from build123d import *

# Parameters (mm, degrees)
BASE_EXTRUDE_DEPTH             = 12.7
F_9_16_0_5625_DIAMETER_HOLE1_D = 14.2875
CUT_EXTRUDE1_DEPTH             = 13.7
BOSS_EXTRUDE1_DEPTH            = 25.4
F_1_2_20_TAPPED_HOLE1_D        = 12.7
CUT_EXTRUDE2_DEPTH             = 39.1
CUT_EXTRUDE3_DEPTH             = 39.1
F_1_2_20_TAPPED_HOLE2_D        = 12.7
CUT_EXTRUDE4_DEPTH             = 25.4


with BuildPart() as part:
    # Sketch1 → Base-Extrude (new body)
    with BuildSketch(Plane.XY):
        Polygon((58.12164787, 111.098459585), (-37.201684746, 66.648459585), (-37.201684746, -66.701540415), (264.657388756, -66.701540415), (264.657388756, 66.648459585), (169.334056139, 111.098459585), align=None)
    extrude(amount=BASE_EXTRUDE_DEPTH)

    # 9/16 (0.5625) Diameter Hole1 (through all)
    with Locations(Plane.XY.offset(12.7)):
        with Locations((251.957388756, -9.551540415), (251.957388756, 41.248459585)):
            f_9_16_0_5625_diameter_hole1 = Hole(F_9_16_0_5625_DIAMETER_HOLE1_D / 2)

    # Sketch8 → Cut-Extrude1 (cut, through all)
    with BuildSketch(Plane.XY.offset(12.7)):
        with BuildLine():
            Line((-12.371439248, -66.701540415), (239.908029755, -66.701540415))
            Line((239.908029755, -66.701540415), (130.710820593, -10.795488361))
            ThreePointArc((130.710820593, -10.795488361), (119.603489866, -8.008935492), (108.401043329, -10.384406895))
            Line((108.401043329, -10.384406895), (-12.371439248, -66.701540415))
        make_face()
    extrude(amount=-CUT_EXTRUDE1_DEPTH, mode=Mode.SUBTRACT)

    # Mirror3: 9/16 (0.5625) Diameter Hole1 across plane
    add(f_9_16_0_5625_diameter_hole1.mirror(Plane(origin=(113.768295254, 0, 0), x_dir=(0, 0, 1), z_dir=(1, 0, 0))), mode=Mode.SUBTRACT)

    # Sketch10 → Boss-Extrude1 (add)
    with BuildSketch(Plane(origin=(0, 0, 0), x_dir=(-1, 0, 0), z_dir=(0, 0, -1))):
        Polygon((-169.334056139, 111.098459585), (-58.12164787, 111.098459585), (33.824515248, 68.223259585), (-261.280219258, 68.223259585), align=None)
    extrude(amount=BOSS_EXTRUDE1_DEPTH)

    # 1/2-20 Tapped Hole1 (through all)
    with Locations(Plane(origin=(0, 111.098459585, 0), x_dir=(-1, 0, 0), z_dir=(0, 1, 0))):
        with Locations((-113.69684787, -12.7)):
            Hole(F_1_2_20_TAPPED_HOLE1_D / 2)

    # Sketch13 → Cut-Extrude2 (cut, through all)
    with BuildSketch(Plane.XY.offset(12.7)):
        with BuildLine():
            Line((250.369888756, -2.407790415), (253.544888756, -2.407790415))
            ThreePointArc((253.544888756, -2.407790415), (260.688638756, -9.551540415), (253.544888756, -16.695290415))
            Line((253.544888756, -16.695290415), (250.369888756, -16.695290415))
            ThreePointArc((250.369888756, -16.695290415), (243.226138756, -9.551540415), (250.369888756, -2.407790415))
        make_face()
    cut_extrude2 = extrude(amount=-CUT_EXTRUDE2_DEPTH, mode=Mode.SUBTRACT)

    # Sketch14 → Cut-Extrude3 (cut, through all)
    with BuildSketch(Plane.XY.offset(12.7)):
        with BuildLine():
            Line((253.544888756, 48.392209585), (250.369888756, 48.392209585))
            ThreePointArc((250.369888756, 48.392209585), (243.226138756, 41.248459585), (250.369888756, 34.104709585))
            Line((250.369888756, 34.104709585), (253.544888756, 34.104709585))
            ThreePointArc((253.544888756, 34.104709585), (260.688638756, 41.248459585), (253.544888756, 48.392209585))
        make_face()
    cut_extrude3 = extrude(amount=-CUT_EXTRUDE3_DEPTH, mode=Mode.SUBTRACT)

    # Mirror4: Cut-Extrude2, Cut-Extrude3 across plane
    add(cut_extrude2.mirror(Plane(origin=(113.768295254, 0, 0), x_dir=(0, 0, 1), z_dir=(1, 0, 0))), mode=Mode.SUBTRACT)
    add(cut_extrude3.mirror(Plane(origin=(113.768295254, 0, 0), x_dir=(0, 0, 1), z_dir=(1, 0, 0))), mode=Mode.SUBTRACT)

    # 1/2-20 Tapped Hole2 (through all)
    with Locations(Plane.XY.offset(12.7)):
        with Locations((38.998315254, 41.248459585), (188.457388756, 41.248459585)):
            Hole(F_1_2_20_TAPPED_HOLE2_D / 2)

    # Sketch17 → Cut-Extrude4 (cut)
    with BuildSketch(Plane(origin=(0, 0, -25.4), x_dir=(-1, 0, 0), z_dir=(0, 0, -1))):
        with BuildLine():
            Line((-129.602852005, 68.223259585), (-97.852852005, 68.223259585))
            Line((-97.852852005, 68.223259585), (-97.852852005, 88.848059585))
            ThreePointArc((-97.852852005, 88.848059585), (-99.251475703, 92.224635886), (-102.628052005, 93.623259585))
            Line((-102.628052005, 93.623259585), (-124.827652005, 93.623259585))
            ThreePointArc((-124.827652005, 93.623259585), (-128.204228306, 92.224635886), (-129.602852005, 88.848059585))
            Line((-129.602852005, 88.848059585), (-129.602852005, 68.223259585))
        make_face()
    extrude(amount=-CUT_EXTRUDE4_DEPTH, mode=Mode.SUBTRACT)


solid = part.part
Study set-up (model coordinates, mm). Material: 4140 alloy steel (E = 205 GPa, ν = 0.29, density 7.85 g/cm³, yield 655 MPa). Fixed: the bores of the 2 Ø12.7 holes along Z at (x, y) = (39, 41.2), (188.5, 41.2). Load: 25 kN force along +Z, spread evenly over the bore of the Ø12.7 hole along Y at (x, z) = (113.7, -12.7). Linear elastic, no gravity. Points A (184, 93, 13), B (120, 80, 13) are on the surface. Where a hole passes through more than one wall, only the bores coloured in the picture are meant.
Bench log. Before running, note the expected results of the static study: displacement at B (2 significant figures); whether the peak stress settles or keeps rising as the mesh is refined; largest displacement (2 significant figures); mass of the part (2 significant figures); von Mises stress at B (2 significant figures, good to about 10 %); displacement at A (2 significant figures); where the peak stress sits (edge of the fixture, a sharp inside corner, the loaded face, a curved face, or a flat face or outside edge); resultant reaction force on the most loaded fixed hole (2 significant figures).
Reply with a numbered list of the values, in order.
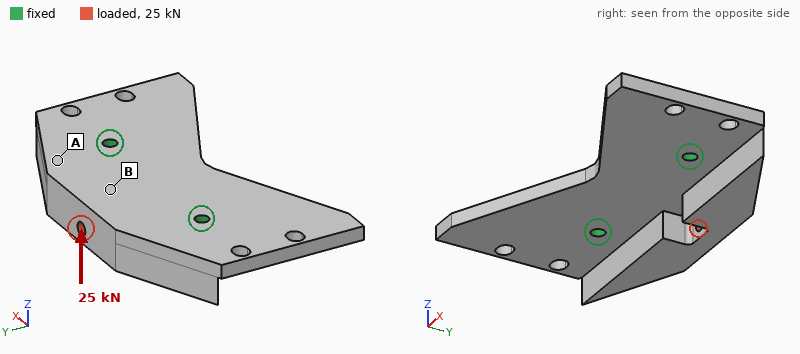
1. 0.22 mm
2. keeps rising
3. 0.46 mm
4. 5.6 kg
5. 80 MPa
6. 0.24 mm
7. edge of the fixture
8. 13 kN
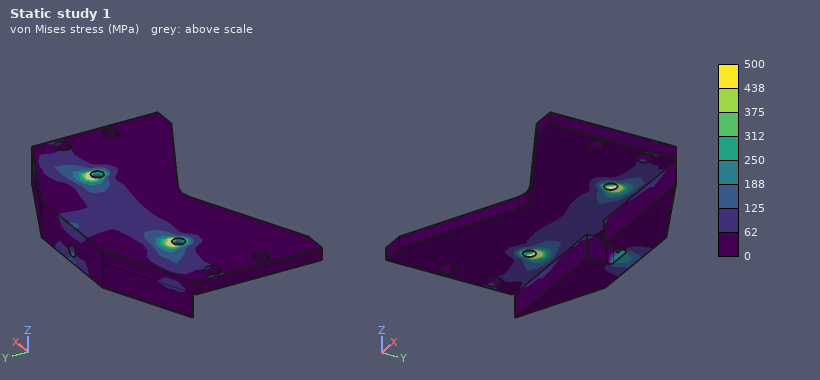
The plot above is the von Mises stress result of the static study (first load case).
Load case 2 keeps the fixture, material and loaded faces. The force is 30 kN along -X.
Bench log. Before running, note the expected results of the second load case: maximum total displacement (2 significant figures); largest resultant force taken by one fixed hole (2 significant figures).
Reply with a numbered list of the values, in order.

1. 26 µm
2. 19 kN
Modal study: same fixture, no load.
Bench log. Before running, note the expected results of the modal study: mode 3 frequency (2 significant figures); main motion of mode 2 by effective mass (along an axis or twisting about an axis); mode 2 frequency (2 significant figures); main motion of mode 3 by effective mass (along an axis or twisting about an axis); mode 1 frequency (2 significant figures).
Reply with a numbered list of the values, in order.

1. 1300 Hz
2. twisting about Y
3. 960 Hz
4. along Z
5. 860 Hz
